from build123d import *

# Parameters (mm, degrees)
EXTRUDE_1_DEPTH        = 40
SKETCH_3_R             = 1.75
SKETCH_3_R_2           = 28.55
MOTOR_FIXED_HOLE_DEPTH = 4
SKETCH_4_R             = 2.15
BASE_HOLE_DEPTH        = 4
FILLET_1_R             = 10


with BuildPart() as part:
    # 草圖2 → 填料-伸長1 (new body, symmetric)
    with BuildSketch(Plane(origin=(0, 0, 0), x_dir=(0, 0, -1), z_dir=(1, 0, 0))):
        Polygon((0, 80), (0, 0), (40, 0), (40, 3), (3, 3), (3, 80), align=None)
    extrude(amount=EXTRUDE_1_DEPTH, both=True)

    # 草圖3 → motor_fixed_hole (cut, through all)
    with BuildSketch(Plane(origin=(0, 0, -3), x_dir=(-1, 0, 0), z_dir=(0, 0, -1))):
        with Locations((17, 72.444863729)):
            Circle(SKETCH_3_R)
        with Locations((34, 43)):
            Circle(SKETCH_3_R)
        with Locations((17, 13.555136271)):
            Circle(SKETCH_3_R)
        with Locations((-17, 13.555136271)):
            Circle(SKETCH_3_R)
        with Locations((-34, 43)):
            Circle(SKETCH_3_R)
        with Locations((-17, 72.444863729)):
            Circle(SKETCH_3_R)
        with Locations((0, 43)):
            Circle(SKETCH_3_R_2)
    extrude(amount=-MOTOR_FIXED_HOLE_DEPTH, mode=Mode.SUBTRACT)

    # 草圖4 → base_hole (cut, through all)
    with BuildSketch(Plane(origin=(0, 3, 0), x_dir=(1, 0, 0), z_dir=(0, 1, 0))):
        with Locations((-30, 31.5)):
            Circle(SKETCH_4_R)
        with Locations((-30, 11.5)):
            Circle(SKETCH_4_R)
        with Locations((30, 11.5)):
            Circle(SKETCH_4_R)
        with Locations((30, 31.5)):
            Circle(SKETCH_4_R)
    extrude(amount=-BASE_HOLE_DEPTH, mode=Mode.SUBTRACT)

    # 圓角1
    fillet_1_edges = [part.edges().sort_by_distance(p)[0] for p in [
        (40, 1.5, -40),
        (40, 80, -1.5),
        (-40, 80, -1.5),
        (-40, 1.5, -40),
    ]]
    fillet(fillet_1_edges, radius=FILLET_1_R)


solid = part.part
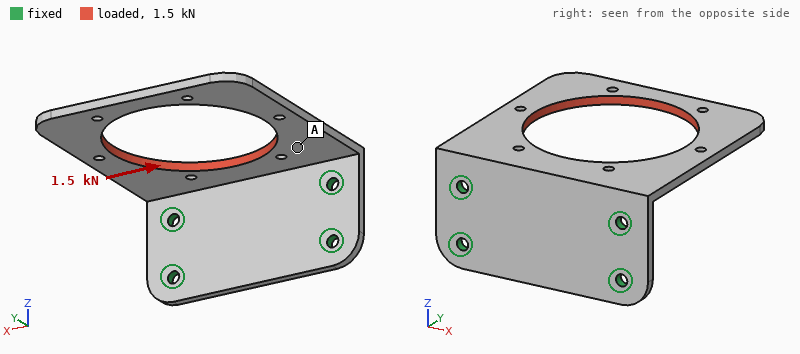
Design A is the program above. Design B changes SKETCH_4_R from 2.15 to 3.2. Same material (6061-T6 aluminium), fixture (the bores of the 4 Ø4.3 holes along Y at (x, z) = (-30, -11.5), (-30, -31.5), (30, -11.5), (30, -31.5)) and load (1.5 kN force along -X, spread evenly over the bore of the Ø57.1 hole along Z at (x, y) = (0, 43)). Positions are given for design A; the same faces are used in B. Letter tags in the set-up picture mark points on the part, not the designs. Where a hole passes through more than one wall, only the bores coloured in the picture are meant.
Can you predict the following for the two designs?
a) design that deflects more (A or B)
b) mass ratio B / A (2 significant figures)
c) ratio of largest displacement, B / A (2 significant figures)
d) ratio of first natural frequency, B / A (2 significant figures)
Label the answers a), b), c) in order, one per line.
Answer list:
a) A
b) 0.99
c) 0.82
d) 1.0
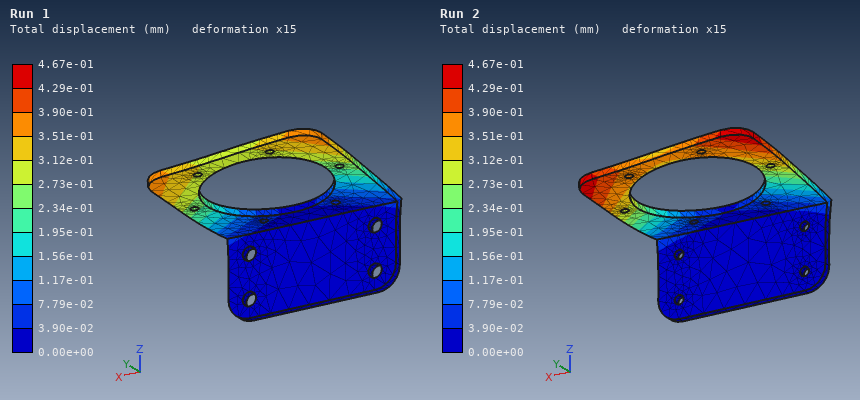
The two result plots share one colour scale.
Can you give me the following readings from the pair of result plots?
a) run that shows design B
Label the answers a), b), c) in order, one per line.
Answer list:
a) Run 1
